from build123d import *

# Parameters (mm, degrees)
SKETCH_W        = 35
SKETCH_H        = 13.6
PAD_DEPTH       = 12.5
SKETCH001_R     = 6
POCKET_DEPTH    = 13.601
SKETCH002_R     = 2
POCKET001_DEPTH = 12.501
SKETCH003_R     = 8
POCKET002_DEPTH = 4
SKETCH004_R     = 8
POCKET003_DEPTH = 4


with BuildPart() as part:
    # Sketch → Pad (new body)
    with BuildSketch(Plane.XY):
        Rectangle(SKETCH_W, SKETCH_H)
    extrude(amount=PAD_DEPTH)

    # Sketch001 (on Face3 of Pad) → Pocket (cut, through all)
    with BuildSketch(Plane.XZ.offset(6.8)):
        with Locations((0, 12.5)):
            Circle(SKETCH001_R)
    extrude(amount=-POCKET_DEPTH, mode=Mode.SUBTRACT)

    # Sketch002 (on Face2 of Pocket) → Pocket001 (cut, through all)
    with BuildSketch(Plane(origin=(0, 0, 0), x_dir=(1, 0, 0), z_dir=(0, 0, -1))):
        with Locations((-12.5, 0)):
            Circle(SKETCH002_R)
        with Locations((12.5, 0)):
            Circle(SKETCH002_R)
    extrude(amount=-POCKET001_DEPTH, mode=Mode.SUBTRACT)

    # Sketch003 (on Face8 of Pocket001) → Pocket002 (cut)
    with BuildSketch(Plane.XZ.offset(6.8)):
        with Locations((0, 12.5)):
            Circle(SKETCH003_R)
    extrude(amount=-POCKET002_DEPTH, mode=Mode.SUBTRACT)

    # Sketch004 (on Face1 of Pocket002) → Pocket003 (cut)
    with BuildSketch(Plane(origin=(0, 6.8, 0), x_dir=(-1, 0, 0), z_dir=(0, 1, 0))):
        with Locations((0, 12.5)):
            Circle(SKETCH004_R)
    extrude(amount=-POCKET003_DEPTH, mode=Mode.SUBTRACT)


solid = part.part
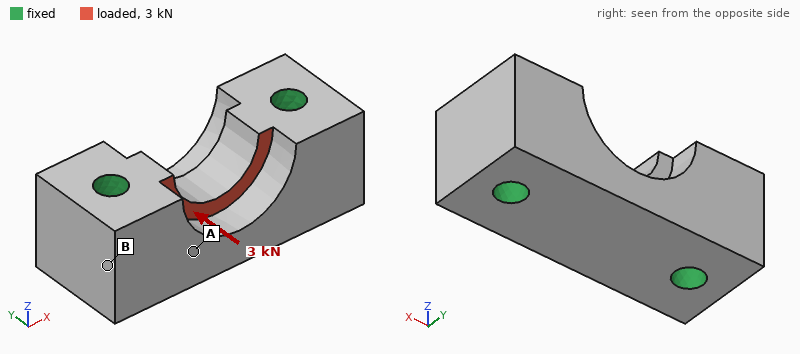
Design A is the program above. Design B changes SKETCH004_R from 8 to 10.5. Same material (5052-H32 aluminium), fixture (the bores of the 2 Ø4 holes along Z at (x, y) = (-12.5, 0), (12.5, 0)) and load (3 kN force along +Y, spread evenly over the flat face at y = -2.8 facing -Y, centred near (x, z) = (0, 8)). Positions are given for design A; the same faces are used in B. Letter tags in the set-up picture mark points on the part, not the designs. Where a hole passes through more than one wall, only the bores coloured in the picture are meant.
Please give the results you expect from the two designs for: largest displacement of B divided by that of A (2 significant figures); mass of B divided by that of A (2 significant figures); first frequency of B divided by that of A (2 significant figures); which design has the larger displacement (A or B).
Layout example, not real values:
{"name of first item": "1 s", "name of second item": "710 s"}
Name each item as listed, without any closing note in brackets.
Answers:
{"largest displacement of B divided by that of A": "1.2", "mass of B divided by that of A": "0.94", "first frequency of B divided by that of A": "1.0", "which design has the larger displacement": "B"}
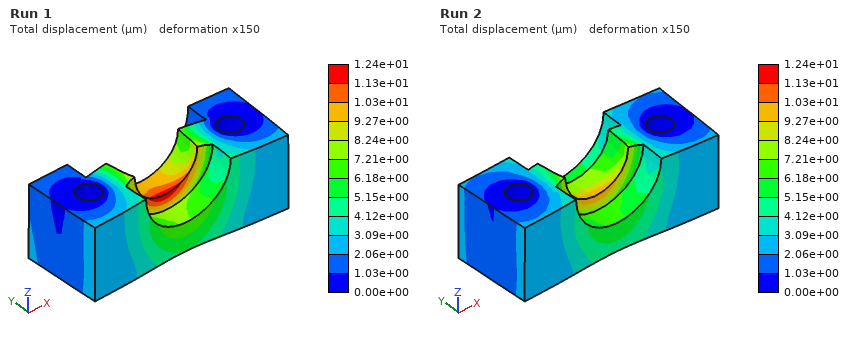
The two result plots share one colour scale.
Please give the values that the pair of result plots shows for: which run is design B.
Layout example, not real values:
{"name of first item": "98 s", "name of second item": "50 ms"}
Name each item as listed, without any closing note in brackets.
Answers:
{"which run is design B": "Run 1"}
